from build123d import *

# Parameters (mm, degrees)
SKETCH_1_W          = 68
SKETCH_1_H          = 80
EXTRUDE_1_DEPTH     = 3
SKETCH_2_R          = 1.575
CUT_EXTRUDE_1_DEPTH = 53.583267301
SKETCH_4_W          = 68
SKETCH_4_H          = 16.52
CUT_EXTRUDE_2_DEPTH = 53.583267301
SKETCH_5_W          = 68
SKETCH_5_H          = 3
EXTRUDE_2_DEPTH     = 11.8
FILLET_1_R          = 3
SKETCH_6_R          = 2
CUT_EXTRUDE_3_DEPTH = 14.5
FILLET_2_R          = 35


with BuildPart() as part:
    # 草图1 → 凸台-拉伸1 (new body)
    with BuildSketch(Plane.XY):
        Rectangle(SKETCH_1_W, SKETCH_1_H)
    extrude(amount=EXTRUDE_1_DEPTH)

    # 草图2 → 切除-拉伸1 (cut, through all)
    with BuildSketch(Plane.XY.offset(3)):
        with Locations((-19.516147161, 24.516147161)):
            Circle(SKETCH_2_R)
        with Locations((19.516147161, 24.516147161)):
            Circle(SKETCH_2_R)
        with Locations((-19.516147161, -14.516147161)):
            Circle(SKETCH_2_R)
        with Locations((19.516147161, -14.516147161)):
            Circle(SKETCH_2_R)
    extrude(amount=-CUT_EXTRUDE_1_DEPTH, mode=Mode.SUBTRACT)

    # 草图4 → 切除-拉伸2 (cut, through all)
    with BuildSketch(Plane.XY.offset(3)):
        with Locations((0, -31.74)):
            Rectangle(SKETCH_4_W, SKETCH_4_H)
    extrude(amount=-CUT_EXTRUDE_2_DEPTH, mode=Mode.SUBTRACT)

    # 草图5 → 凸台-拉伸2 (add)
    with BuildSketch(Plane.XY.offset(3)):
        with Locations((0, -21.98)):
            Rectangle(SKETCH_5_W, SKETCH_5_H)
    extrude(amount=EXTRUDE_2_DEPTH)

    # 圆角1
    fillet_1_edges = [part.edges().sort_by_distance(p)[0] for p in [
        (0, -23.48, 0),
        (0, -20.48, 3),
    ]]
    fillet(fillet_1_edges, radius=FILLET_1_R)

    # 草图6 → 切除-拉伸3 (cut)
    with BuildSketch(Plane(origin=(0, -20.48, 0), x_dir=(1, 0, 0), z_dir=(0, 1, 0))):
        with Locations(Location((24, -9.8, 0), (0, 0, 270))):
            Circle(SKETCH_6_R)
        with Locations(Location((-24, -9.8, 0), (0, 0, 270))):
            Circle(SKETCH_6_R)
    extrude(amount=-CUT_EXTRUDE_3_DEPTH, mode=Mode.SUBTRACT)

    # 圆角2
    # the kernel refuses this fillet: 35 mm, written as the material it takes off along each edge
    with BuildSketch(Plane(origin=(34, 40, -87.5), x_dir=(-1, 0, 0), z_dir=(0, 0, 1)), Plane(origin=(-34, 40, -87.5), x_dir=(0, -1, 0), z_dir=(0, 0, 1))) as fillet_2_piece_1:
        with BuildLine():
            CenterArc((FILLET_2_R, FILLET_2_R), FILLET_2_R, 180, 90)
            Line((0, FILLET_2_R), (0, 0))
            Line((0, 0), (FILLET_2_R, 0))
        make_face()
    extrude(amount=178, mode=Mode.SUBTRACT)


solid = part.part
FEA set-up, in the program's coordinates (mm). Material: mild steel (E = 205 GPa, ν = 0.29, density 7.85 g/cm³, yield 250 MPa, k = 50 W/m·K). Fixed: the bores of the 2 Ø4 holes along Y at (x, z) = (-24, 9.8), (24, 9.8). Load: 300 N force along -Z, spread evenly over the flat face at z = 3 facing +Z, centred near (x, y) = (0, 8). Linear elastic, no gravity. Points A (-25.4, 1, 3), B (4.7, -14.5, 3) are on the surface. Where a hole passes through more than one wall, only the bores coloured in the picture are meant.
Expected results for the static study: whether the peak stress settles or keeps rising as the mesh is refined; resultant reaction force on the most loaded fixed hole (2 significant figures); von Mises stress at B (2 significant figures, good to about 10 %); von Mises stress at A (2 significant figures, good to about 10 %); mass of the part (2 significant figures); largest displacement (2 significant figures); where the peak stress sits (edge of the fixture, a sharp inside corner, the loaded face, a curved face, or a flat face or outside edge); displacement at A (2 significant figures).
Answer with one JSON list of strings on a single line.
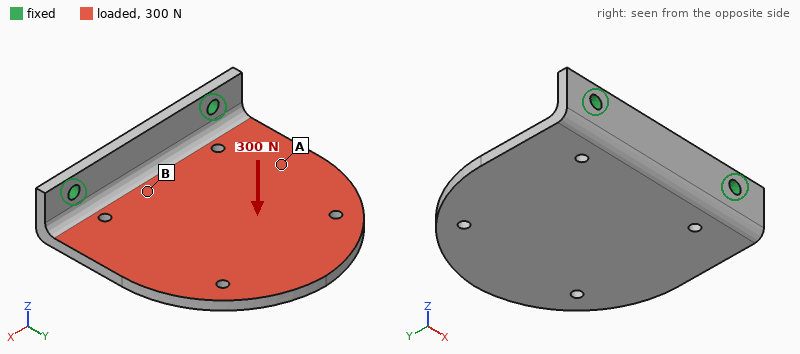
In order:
["keeps rising", "170 N", "57 MPa", "29 MPa", "110 g", "0.40 mm", "edge of the fixture", "0.11 mm"]
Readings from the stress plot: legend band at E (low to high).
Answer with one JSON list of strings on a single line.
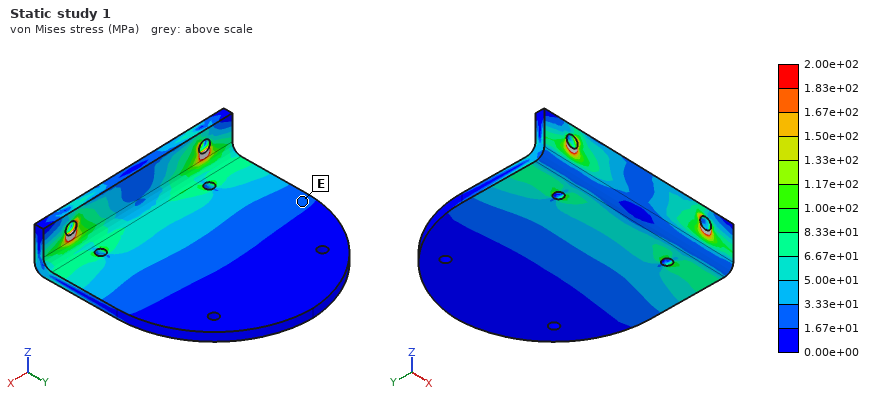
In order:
["1.67e+01 to 3.33e+01 MPa"]
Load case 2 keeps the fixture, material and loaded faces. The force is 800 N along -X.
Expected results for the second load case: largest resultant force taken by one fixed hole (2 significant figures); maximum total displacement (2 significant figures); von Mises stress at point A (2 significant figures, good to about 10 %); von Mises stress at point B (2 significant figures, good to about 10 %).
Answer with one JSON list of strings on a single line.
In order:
["630 N", "39 µm", "15 MPa", "23 MPa"]
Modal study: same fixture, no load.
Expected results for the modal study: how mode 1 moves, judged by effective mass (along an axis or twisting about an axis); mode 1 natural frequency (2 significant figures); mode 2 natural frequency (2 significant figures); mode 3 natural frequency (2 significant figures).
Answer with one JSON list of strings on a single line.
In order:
["along Z", "640 Hz", "1900 Hz", "3500 Hz"]
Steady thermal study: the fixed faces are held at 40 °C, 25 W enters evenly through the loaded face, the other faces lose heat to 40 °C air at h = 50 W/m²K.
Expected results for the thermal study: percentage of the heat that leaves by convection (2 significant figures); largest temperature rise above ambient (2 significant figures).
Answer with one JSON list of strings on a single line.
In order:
["46 %", "62 K"]
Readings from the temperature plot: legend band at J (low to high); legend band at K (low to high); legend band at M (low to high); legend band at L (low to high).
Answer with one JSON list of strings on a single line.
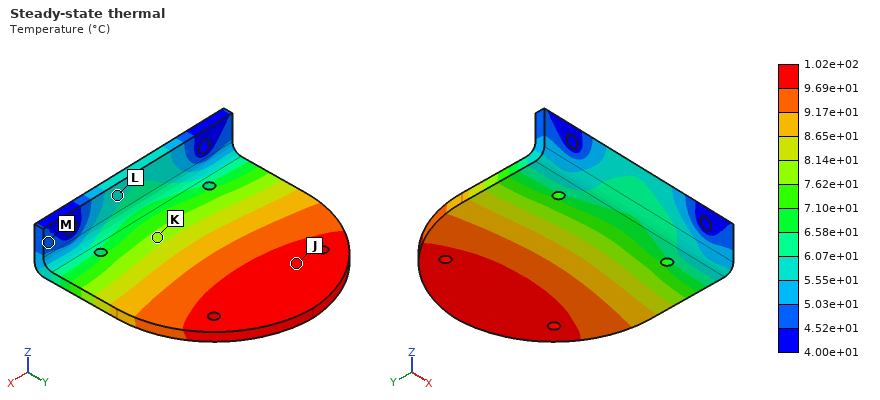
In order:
["9.69e+01 to 1.02e+02 °C", "7.62e+01 to 8.14e+01 °C", "4.52e+01 to 5.03e+01 °C", "5.55e+01 to 6.07e+01 °C"]
